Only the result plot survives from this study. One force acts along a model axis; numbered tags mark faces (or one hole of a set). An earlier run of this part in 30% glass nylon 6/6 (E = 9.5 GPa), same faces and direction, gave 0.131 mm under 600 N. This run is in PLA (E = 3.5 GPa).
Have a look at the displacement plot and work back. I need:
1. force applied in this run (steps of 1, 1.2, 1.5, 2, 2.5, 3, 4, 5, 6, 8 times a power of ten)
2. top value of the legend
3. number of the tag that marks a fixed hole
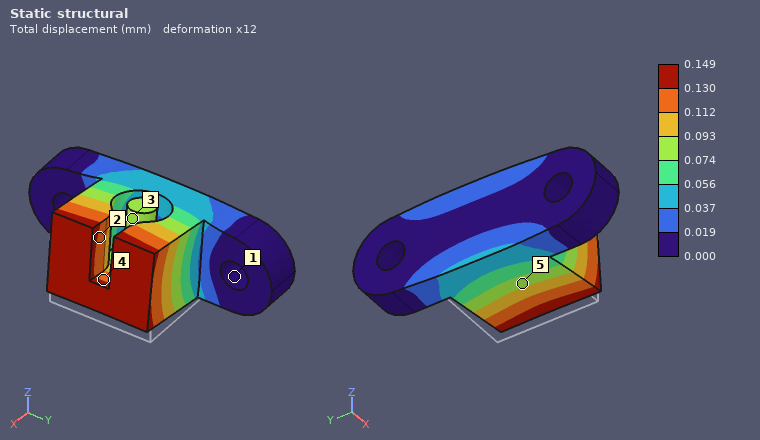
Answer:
250 N
0.149 mm
1
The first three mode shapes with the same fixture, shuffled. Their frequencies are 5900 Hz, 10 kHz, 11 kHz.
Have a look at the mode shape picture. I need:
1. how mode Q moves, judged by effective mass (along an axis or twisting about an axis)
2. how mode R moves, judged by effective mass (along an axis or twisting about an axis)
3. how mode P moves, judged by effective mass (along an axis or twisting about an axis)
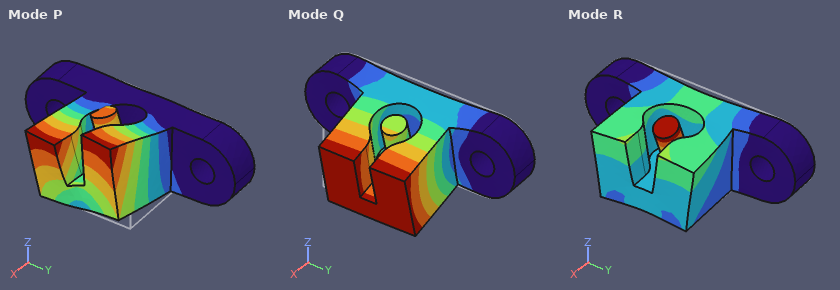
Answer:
along Z
along X
along Y
